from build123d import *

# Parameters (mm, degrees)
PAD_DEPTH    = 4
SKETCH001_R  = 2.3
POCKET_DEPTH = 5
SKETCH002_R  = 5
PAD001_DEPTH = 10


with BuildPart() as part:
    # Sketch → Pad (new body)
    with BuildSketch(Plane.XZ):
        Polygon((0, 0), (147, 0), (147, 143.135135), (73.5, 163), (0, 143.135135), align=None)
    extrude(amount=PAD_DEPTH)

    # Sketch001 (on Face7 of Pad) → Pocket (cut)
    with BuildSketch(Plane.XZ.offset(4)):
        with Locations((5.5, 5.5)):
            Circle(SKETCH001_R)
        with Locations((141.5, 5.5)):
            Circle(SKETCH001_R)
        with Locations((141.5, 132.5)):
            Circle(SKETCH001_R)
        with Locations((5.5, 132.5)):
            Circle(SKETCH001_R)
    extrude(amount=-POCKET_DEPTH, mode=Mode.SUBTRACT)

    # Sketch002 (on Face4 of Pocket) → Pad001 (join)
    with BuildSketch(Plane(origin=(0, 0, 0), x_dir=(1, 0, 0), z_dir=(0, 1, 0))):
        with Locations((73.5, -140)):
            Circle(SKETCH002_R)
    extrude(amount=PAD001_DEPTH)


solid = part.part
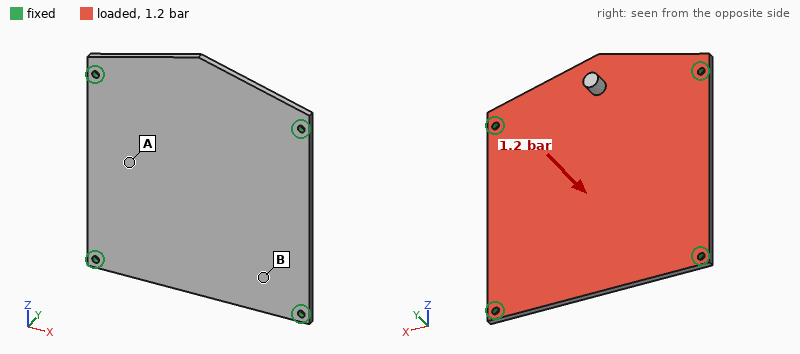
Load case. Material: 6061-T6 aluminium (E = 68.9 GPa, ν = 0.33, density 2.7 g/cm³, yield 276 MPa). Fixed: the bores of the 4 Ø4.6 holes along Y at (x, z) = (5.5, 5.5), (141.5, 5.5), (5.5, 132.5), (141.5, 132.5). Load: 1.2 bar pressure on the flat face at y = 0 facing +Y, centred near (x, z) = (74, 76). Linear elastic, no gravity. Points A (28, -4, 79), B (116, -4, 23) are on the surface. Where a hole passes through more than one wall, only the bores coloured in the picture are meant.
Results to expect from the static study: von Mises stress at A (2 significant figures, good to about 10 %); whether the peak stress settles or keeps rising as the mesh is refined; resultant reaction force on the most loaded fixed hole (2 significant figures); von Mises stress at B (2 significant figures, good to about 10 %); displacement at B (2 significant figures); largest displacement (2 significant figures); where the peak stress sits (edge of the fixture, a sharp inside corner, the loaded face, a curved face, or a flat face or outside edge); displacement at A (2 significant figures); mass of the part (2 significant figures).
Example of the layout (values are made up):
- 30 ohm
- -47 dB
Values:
- 39 MPa
- keeps rising
- 750 N
- 17 MPa
- 0.34 mm
- 0.78 mm
- edge of the fixture
- 0.54 mm
- 240 g
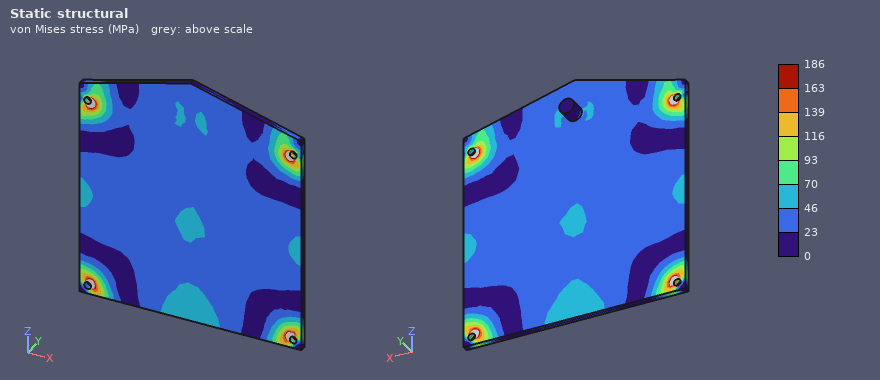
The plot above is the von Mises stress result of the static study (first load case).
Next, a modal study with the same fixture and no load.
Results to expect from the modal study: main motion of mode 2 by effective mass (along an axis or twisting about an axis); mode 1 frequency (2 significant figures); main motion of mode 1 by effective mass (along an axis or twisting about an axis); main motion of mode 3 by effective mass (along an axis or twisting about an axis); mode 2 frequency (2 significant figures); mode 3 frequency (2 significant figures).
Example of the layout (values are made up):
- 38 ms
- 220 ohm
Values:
- twisting about X
- 720 Hz
- along Y
- twisting about Z
- 1100 Hz
- 1300 Hz
